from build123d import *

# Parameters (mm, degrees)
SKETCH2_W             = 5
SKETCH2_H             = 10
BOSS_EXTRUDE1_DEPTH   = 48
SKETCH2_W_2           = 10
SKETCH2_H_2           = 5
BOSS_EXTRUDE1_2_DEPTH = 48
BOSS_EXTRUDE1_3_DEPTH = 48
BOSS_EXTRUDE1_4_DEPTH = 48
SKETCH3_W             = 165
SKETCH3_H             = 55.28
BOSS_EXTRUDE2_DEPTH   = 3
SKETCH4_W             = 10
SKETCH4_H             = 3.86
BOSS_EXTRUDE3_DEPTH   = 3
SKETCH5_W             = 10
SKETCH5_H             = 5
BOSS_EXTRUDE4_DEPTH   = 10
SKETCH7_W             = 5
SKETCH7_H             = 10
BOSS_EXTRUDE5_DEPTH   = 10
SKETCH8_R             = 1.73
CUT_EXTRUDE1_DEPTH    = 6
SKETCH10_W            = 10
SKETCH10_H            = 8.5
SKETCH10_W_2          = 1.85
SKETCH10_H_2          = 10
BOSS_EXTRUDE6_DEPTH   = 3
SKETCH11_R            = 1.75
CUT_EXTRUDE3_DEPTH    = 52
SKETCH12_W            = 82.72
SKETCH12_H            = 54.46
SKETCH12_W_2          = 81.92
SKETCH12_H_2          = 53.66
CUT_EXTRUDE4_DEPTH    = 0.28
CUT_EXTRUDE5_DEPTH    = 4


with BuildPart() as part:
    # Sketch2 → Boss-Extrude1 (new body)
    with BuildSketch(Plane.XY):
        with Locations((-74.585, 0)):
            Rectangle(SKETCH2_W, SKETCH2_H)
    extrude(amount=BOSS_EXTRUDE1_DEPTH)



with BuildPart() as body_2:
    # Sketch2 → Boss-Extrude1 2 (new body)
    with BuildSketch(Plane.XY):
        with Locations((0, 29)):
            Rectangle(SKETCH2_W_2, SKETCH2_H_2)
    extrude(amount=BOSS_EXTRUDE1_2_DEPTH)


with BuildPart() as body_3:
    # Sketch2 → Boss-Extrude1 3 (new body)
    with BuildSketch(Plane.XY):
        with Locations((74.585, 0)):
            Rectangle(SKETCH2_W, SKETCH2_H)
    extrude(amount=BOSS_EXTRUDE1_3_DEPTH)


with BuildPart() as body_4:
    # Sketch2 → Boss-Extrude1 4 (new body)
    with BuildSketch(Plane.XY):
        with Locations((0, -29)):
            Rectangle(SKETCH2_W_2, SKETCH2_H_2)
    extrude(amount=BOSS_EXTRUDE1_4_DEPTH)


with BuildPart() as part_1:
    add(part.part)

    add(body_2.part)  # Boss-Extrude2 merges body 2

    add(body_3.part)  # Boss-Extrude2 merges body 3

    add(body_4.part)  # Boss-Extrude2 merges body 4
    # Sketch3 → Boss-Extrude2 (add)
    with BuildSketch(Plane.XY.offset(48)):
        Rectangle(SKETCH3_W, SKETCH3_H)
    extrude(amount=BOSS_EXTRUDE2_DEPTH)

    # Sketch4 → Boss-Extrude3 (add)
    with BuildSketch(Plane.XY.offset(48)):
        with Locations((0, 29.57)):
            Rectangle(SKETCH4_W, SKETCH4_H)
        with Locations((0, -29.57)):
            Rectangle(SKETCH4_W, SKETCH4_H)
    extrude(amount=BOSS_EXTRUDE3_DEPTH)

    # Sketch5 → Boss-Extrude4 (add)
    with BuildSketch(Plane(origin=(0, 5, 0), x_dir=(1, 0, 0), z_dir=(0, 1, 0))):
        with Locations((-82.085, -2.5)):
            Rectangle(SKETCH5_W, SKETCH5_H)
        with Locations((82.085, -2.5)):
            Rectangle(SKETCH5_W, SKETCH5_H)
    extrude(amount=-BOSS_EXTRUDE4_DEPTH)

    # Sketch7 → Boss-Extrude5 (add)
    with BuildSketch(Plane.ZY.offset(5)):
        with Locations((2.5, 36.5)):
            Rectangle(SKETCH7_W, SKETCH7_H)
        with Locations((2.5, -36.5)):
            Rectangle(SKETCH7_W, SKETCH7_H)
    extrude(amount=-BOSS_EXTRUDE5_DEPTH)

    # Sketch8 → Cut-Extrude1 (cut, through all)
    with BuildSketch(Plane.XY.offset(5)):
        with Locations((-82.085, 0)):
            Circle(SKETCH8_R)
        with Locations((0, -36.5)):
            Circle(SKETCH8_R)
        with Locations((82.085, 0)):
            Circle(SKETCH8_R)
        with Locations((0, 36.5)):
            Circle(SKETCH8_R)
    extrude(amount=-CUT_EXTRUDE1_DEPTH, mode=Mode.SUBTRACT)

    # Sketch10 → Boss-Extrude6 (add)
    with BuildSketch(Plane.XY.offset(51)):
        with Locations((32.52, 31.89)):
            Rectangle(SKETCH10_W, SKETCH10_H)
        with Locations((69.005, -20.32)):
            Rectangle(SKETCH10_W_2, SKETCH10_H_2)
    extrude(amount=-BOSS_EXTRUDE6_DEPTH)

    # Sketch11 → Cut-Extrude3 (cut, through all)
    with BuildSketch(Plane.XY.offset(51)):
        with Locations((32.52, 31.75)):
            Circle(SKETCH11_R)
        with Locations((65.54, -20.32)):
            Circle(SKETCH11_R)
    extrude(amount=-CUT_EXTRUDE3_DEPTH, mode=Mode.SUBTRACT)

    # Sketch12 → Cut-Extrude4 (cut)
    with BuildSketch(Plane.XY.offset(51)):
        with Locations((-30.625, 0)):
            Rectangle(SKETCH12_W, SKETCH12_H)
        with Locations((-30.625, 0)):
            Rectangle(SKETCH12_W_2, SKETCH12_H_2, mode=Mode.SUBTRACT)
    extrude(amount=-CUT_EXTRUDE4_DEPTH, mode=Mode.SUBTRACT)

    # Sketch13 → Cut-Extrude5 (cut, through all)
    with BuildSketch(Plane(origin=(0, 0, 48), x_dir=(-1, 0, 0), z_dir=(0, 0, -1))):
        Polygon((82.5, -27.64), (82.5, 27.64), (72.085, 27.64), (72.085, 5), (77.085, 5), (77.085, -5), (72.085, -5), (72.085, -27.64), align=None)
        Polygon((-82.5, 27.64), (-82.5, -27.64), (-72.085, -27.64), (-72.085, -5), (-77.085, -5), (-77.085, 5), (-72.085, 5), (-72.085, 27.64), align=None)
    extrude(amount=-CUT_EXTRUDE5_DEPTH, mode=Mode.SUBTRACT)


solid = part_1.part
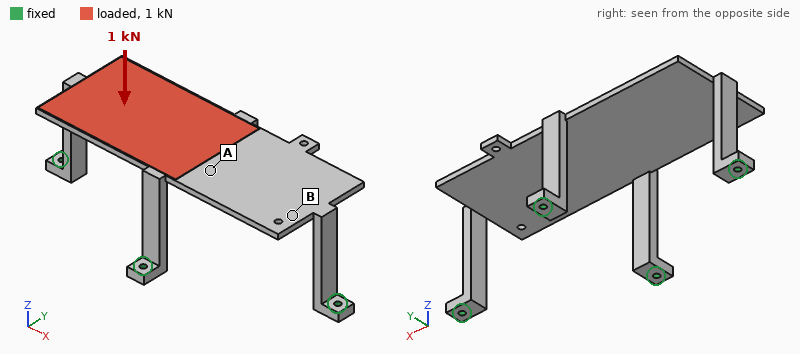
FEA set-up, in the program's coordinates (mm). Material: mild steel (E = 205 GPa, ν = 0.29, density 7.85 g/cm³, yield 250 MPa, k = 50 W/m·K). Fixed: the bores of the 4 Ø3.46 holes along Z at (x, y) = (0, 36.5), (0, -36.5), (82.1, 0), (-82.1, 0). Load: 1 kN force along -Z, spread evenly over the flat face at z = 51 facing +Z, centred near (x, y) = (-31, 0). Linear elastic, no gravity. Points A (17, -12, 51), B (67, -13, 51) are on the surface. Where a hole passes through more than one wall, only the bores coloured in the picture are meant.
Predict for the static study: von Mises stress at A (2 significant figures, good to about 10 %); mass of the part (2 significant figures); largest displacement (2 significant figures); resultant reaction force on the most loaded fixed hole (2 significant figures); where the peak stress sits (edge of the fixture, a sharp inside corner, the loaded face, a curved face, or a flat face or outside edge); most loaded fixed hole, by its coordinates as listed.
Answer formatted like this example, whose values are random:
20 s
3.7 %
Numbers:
17 MPa
280 g
92 µm
400 N
a flat face or outside edge
(-82.1, 0)
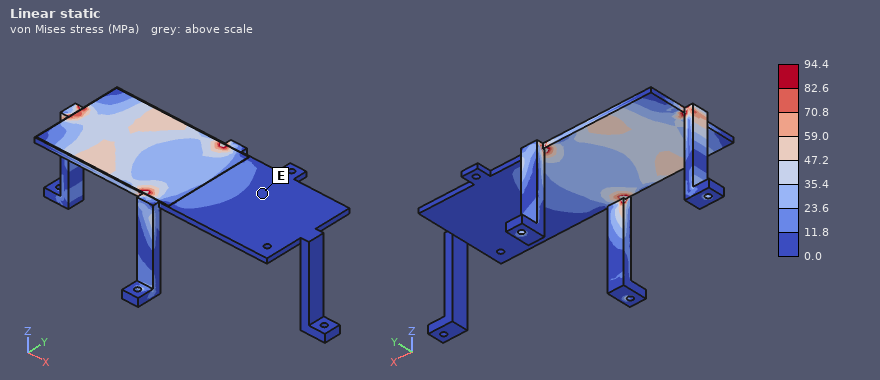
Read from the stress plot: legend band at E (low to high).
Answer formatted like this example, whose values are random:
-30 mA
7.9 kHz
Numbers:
0.0 to 11.8 MPa
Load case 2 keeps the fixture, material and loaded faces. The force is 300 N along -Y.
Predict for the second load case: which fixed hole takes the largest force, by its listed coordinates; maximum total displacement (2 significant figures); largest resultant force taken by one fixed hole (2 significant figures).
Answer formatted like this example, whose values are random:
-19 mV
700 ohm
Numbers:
(-82.1, 0)
99 µm
130 N
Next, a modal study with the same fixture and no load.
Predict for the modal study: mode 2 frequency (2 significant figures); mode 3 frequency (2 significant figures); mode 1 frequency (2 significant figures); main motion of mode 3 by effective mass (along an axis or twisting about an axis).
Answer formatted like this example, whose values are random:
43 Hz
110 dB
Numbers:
810 Hz
1100 Hz
780 Hz
twisting about Z
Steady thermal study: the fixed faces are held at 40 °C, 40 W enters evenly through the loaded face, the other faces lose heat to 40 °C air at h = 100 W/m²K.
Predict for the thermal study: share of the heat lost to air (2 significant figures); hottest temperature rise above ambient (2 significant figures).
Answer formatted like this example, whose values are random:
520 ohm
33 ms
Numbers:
94 %
53 K
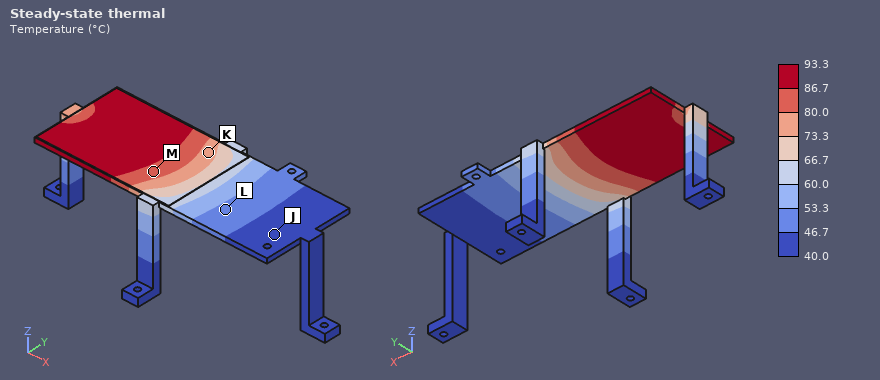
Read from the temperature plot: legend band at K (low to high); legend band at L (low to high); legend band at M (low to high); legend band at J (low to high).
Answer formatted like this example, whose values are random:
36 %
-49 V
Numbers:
73.3 to 80.0 °C
46.7 to 53.3 °C
80.0 to 86.7 °C
40.0 to 46.7 °C
